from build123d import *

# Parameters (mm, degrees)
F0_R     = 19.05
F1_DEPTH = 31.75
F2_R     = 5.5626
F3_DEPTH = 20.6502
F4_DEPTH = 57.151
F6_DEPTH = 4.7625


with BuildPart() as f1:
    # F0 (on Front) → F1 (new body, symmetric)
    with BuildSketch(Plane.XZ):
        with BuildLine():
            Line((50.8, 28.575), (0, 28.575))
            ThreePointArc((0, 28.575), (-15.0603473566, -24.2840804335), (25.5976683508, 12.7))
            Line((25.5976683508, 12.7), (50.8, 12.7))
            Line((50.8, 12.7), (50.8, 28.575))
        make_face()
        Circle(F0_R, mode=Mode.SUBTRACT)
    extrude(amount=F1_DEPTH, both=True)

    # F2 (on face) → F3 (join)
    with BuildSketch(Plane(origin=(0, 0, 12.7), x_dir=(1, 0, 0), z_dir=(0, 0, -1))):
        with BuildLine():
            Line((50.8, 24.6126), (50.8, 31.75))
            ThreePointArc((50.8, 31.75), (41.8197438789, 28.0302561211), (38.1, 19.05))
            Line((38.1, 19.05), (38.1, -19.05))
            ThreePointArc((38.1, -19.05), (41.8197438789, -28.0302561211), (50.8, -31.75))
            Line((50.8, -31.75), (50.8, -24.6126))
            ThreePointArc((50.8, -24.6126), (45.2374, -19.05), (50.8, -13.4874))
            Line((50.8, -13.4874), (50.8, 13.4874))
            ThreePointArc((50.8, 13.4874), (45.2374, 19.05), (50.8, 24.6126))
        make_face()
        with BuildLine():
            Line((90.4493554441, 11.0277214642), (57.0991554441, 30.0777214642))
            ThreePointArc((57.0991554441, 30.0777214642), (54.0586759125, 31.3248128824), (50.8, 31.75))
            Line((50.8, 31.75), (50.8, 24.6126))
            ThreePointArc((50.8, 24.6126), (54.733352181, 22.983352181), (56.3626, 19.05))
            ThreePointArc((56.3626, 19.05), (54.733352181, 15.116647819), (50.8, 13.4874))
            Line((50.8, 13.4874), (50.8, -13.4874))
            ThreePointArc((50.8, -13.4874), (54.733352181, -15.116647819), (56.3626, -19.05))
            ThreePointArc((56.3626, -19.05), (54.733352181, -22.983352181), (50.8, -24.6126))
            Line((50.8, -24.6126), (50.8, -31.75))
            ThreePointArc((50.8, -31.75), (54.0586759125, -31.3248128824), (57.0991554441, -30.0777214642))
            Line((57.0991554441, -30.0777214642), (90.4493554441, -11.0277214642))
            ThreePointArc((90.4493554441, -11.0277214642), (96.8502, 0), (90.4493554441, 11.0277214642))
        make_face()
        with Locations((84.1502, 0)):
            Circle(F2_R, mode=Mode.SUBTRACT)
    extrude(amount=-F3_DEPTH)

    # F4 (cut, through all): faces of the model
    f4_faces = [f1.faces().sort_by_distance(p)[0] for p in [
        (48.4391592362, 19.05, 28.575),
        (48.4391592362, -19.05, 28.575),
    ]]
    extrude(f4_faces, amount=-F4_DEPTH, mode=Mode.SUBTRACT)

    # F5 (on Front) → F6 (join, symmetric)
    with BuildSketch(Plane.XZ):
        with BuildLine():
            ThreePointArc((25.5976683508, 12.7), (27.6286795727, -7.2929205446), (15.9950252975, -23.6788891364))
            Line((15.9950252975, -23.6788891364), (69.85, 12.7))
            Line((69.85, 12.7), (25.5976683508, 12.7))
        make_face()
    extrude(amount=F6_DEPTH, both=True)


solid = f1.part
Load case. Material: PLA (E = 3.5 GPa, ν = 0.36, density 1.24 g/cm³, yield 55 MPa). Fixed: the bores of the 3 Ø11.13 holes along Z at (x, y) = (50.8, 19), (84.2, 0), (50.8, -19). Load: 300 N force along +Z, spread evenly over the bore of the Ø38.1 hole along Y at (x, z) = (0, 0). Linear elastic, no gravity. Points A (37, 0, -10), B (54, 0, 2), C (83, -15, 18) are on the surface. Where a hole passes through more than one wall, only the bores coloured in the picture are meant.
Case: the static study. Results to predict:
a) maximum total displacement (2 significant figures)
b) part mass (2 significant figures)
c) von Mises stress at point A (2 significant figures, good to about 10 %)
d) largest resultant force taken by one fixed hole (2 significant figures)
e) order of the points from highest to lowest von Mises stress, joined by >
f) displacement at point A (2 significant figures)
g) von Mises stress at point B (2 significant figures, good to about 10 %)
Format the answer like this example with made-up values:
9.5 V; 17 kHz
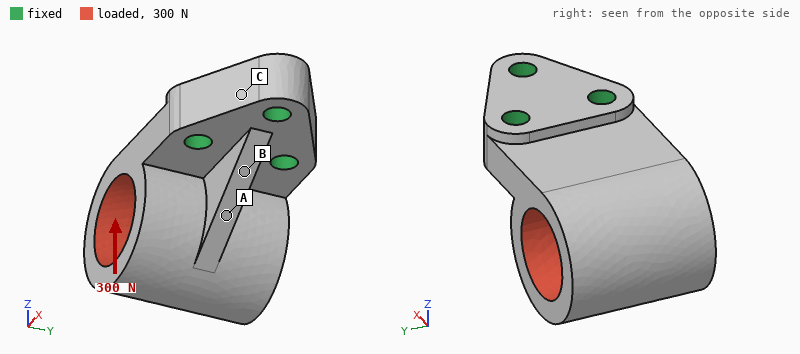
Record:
0.17 mm; 200 g; 1.9 MPa; 210 N; B > A > C; 0.048 mm; 2.7 MPa
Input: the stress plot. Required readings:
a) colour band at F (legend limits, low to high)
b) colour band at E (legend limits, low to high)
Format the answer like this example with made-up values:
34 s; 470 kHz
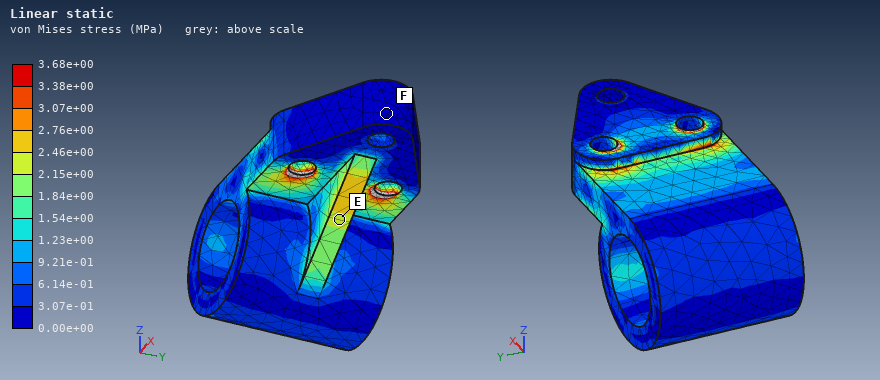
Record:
0.00e+00 to 3.07e-01 MPa; 2.15e+00 to 2.46e+00 MPa
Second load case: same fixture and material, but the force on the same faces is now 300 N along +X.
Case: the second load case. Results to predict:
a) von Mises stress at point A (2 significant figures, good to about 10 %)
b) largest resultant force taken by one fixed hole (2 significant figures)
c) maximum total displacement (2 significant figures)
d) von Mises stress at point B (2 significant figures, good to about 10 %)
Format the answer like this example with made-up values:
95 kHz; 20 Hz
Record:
1.8 MPa; 120 N; 83 µm; 1.7 MPa
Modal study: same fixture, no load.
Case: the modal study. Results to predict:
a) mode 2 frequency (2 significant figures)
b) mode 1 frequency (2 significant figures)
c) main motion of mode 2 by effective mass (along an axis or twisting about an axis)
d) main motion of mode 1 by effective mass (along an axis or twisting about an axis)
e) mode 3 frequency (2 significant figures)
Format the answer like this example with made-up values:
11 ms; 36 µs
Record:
1100 Hz; 670 Hz; along Y; along Z; 1900 Hz
